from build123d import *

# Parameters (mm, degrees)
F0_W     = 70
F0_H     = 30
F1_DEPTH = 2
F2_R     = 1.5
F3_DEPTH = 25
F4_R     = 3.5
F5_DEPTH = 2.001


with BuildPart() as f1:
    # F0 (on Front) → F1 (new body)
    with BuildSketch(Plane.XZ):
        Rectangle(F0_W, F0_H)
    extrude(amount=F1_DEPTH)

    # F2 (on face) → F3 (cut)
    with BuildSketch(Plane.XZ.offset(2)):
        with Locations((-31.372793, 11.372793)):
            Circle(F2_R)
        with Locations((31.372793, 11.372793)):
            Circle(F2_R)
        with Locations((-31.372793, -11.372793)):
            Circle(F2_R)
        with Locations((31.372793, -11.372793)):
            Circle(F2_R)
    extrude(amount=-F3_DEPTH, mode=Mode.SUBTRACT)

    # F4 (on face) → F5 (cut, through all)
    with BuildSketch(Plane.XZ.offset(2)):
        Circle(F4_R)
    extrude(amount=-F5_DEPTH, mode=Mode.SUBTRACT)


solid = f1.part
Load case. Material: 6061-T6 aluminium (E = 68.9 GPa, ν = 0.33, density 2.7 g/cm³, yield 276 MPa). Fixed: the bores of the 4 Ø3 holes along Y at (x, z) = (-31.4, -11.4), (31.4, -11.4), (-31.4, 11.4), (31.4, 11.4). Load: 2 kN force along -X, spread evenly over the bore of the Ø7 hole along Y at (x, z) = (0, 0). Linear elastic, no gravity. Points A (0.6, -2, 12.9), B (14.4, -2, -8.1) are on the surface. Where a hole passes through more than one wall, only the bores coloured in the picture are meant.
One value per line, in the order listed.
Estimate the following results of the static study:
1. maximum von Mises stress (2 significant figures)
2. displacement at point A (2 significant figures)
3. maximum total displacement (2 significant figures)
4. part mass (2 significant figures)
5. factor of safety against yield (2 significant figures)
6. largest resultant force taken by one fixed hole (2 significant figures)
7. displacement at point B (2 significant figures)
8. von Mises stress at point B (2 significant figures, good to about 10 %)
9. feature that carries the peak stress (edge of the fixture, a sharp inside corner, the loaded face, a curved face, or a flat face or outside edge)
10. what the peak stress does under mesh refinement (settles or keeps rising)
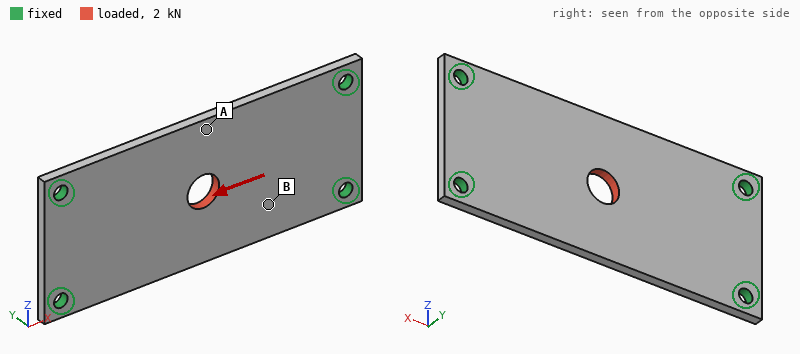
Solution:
78 MPa
6.1 µm
12 µm
11 g
3.5
510 N
5.6 µm
19 MPa
the loaded face
settles
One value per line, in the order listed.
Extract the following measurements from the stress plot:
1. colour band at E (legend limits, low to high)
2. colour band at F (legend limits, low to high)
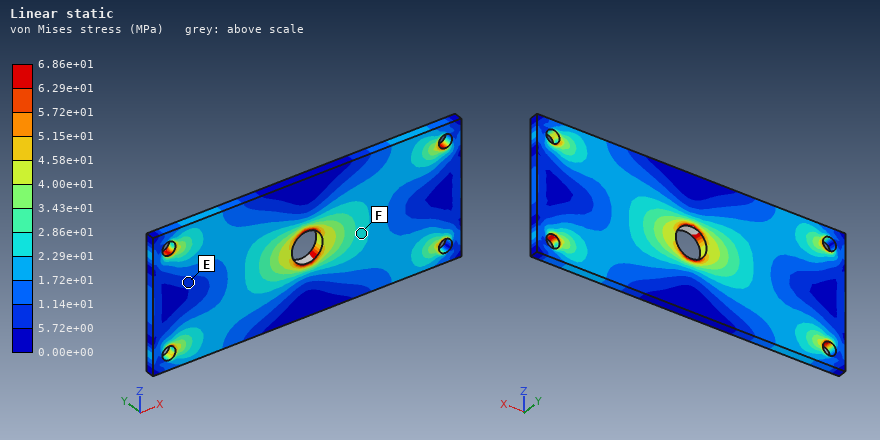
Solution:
5.72e+00 to 1.14e+01 MPa
2.29e+01 to 2.86e+01 MPa
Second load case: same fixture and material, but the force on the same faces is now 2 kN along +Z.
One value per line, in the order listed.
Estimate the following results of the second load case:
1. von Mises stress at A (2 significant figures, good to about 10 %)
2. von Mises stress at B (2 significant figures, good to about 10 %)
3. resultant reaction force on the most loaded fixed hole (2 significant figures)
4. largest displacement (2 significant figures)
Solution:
43 MPa
32 MPa
820 N
33 µm
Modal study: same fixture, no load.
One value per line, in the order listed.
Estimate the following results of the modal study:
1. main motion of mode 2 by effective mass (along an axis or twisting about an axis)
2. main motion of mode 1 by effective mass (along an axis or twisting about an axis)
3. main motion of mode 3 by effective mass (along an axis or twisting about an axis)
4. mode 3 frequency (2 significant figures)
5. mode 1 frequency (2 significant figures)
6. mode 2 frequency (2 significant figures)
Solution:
twisting about X
along Y
twisting about Z
7100 Hz
2600 Hz
4600 Hz
